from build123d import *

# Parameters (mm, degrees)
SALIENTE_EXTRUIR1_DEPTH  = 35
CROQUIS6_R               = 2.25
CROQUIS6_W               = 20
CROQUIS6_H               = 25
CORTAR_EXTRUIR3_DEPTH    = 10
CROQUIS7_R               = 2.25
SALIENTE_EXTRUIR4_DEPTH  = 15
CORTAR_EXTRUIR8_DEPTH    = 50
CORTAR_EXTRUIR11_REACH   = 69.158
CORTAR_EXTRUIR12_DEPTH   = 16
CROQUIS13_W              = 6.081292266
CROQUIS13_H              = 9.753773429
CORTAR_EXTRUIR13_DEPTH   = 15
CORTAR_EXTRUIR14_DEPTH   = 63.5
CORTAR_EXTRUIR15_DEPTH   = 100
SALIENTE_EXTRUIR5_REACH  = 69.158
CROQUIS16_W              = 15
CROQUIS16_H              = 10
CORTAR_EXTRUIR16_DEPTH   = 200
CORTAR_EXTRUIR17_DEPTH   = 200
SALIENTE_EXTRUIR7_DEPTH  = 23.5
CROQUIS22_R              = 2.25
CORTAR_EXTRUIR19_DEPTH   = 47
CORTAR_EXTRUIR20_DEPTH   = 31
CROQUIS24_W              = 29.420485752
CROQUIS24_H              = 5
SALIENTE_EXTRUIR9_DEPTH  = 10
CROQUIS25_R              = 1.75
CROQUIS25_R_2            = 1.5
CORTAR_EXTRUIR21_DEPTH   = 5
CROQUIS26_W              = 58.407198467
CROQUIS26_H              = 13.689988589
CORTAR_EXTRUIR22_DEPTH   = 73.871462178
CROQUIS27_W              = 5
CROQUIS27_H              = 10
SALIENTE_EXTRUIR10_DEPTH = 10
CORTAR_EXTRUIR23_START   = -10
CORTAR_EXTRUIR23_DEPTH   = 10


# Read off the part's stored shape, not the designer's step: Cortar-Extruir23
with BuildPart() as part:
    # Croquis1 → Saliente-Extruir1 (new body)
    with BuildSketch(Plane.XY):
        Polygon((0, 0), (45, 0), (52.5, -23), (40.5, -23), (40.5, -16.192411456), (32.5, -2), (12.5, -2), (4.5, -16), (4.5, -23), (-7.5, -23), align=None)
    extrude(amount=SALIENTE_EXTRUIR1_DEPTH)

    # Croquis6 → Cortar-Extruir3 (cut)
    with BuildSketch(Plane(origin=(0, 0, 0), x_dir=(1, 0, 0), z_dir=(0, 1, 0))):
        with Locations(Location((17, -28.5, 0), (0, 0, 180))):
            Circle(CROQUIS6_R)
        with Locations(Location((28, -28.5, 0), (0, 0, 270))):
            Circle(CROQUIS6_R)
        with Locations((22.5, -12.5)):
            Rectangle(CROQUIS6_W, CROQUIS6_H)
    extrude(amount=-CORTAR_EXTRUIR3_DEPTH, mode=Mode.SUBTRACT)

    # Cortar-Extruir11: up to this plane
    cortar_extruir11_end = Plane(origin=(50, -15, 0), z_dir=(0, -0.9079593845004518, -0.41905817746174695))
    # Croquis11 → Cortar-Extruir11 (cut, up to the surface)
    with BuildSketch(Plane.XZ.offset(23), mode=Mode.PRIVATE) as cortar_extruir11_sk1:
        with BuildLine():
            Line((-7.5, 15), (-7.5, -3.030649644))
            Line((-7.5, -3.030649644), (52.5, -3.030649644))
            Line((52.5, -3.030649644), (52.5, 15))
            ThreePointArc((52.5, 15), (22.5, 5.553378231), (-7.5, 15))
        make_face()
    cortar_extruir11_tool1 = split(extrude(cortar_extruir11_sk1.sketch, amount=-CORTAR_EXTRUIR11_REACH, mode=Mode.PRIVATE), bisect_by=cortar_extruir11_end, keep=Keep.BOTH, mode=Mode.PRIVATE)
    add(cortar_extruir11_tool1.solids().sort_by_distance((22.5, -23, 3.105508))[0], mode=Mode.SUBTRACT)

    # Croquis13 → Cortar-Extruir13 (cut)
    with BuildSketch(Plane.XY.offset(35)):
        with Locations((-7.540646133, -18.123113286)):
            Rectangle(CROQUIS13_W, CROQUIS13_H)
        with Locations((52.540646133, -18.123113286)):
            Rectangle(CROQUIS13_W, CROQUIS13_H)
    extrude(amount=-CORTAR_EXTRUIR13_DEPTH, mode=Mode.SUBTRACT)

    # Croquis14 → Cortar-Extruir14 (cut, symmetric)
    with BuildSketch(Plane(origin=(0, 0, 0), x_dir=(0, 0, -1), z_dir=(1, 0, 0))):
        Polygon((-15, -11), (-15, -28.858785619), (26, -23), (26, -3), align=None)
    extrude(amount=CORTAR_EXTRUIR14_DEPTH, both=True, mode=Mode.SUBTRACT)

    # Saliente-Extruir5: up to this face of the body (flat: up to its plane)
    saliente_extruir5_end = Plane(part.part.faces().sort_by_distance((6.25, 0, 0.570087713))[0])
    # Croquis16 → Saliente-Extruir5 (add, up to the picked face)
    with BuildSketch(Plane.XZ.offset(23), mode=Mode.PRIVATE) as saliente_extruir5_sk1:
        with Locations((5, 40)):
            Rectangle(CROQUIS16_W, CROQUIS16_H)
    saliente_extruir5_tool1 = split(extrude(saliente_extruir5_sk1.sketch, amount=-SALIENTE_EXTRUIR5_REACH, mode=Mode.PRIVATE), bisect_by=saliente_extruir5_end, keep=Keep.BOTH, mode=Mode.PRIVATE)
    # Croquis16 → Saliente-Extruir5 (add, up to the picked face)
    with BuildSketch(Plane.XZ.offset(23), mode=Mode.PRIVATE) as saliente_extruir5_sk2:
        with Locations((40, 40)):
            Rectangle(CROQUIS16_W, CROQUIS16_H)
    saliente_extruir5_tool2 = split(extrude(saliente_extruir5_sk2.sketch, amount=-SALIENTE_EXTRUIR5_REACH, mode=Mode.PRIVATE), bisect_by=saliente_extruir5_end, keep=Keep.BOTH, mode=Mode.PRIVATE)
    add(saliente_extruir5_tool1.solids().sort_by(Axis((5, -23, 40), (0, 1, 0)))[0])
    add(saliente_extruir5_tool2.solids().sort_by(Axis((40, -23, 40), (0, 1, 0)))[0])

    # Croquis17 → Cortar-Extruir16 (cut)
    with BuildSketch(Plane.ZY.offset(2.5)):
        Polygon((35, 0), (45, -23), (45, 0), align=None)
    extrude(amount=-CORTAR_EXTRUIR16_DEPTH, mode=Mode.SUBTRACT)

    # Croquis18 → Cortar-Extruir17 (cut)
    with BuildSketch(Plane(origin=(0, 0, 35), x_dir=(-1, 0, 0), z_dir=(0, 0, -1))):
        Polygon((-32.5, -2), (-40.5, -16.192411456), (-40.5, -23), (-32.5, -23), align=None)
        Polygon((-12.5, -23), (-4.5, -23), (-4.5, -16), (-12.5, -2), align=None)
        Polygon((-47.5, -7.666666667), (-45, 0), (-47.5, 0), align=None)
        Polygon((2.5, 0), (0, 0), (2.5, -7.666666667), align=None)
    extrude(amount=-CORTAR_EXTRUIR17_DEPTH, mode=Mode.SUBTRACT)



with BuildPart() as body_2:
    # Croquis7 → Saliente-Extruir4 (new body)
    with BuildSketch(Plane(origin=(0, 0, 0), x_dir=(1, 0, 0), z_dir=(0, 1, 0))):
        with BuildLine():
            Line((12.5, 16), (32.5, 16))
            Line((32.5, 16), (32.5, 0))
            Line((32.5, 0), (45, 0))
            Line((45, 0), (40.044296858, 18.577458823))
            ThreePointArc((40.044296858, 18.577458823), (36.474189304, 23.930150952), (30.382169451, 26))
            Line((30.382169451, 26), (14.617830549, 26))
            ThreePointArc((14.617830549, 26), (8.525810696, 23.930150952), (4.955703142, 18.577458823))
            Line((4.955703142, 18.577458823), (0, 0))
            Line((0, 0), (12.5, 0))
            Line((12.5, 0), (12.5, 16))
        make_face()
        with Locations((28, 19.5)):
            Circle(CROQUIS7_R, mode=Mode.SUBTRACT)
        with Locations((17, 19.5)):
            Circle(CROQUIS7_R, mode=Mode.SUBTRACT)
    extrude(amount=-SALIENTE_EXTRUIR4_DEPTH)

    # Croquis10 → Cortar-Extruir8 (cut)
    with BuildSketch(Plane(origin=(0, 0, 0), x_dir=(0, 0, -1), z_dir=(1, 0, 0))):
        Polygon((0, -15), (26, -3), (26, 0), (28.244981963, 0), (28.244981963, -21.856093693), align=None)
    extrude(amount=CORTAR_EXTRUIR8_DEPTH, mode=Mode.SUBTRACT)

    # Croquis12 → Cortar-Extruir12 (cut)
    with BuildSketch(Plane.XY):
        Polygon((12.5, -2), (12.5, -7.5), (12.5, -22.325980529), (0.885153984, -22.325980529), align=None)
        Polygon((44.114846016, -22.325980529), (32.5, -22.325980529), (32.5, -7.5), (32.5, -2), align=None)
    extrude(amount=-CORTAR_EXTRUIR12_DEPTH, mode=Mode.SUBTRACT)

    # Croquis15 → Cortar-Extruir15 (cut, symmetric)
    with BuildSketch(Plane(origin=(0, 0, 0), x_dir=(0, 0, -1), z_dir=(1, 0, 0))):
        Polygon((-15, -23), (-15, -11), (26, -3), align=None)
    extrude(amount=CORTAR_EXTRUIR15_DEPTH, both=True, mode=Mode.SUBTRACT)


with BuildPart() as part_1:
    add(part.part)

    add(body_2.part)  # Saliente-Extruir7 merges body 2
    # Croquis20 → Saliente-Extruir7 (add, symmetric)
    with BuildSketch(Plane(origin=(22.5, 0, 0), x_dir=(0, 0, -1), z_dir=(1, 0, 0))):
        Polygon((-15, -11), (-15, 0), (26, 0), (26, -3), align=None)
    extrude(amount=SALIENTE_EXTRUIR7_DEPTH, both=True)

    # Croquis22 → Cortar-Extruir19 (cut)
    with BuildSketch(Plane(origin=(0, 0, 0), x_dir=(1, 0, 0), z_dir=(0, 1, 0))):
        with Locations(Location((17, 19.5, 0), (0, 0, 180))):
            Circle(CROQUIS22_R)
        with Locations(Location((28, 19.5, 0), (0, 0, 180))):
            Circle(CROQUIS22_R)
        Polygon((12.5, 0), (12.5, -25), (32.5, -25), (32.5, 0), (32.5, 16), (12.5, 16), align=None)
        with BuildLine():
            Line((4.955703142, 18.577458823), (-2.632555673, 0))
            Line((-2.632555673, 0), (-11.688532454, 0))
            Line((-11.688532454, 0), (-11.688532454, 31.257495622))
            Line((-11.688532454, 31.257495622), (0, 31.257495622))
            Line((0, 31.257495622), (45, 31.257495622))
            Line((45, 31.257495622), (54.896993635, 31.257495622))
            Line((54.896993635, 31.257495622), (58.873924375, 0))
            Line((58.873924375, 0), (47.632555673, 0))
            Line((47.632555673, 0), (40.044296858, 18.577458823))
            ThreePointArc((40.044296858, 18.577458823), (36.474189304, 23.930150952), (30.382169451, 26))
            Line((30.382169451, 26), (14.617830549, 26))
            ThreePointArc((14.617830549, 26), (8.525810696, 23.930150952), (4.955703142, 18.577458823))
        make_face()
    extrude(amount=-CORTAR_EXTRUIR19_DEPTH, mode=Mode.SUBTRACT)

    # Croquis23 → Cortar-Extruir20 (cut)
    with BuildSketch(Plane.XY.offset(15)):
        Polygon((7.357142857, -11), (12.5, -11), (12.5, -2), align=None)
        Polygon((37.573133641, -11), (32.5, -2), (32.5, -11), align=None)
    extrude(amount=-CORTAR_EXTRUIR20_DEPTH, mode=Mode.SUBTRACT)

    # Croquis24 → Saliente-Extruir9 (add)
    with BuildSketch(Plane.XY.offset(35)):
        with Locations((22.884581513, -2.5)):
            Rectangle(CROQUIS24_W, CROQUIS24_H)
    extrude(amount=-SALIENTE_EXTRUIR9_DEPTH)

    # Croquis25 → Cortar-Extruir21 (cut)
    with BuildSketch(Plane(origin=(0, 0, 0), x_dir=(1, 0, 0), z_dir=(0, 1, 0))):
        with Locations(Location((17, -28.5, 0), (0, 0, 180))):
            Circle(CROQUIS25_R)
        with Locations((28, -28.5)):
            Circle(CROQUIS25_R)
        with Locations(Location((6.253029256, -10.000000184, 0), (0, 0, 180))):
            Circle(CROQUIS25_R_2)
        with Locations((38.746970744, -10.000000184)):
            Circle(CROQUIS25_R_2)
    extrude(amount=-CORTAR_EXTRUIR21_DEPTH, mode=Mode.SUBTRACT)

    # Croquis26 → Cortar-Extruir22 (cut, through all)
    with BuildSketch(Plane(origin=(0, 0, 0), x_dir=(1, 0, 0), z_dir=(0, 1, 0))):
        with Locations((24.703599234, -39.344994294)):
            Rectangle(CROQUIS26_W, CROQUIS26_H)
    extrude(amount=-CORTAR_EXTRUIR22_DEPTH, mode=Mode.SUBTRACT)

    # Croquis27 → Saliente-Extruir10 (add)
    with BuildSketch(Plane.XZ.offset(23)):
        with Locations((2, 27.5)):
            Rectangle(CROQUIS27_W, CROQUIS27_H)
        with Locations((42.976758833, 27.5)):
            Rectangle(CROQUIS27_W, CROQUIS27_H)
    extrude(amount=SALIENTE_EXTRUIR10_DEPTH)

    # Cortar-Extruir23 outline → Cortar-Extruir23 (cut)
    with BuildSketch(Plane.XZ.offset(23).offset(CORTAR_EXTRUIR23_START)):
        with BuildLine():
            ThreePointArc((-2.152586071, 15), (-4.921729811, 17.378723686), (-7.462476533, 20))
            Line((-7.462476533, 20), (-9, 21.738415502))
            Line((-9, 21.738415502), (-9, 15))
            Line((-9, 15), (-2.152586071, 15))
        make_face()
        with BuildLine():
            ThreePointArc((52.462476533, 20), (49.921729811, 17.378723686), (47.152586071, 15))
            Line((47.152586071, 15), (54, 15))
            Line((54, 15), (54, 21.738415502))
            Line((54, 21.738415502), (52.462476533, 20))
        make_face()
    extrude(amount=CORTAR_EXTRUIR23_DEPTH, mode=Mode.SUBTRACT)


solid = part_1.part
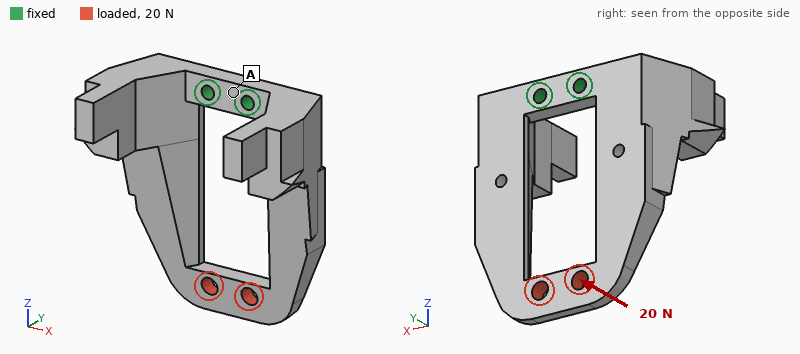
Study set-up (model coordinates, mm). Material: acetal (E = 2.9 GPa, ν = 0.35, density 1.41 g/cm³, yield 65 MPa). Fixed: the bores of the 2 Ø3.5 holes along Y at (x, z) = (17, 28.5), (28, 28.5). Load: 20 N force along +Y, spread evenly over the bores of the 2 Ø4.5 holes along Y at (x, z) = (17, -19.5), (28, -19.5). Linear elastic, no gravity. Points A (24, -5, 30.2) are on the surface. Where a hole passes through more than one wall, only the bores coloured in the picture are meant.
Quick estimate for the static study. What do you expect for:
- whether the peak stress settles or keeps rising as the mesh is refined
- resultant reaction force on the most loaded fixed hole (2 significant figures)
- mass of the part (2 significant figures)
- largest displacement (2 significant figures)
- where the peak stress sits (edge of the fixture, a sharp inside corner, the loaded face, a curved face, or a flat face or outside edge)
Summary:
keeps rising
10 N
24 g
0.99 mm
edge of the fixture
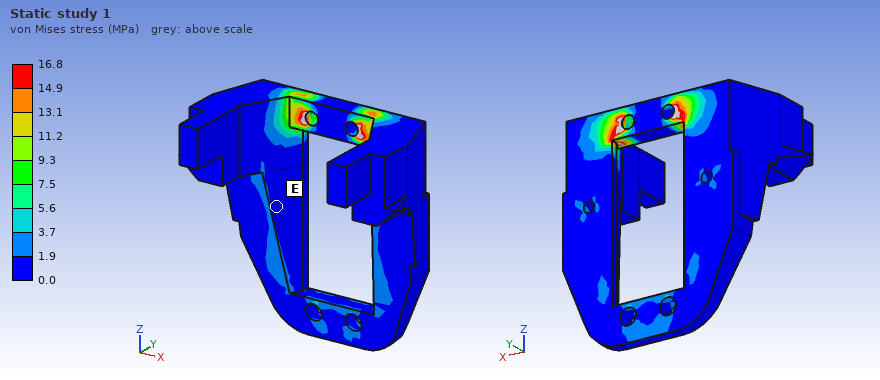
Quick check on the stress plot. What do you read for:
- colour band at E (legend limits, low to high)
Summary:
0.0 to 1.9 MPa
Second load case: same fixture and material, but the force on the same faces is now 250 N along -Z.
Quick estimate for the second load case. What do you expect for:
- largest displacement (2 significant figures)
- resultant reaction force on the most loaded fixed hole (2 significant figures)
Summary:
0.28 mm
130 N
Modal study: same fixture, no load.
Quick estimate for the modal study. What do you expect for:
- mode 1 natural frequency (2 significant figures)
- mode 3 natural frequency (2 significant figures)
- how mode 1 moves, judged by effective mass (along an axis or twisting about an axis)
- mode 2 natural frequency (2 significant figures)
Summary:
340 Hz
510 Hz
along Y
500 Hz
